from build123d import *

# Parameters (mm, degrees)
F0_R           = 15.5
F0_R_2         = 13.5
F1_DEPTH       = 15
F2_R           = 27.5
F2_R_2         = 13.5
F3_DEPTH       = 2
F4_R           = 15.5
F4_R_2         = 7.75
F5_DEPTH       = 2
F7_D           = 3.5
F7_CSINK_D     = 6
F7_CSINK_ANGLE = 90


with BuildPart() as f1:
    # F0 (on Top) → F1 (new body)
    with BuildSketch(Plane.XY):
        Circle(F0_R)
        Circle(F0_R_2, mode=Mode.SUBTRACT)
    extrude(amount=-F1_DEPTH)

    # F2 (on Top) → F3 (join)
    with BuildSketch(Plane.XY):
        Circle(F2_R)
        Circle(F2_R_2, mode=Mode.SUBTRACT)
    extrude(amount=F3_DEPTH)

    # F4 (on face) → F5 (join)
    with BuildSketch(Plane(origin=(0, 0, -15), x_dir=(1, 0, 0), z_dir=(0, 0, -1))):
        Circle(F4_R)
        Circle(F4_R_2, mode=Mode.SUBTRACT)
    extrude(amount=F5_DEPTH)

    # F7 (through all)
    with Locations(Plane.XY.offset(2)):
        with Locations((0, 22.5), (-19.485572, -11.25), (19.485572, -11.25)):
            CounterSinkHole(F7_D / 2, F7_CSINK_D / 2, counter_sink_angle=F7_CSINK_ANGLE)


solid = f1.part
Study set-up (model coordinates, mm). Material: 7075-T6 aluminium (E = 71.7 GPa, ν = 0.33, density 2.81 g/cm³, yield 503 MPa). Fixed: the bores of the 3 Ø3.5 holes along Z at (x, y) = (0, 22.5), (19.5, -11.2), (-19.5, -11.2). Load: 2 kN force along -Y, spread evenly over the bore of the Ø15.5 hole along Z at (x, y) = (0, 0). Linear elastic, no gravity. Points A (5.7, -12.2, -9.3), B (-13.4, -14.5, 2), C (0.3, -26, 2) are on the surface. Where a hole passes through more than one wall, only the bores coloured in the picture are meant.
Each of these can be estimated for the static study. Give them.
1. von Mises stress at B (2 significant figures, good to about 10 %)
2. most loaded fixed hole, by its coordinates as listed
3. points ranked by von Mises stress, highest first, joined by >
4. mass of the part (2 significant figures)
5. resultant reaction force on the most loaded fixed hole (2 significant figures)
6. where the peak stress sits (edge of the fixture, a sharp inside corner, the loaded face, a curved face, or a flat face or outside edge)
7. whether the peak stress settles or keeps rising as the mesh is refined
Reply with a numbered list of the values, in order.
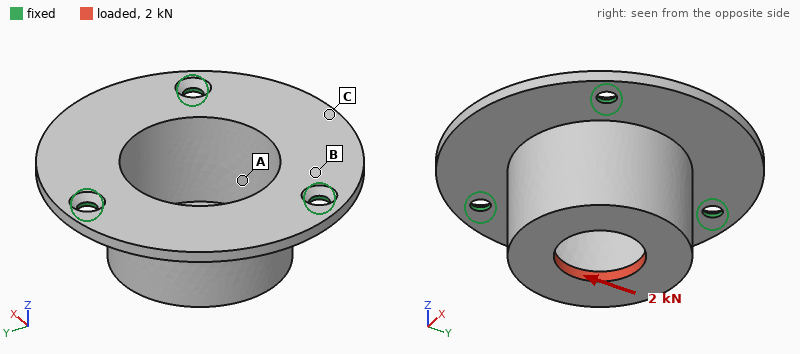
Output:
1. 91 MPa
2. (0, 22.5)
3. B > C > A
4. 21 g
5. 1.2 kN
6. edge of the fixture
7. keeps rising
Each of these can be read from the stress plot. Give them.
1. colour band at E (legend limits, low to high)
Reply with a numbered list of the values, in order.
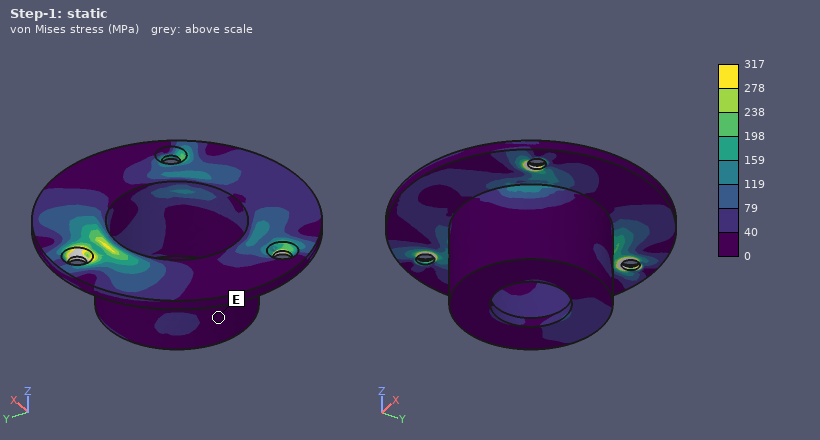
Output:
1. 0 to 40 MPa
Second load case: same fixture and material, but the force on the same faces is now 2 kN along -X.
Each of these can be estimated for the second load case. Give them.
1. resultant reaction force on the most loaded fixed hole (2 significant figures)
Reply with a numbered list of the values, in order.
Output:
1. 1.1 kN
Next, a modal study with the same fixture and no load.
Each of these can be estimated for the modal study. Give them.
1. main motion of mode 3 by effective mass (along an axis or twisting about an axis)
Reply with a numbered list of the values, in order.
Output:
1. along Z
